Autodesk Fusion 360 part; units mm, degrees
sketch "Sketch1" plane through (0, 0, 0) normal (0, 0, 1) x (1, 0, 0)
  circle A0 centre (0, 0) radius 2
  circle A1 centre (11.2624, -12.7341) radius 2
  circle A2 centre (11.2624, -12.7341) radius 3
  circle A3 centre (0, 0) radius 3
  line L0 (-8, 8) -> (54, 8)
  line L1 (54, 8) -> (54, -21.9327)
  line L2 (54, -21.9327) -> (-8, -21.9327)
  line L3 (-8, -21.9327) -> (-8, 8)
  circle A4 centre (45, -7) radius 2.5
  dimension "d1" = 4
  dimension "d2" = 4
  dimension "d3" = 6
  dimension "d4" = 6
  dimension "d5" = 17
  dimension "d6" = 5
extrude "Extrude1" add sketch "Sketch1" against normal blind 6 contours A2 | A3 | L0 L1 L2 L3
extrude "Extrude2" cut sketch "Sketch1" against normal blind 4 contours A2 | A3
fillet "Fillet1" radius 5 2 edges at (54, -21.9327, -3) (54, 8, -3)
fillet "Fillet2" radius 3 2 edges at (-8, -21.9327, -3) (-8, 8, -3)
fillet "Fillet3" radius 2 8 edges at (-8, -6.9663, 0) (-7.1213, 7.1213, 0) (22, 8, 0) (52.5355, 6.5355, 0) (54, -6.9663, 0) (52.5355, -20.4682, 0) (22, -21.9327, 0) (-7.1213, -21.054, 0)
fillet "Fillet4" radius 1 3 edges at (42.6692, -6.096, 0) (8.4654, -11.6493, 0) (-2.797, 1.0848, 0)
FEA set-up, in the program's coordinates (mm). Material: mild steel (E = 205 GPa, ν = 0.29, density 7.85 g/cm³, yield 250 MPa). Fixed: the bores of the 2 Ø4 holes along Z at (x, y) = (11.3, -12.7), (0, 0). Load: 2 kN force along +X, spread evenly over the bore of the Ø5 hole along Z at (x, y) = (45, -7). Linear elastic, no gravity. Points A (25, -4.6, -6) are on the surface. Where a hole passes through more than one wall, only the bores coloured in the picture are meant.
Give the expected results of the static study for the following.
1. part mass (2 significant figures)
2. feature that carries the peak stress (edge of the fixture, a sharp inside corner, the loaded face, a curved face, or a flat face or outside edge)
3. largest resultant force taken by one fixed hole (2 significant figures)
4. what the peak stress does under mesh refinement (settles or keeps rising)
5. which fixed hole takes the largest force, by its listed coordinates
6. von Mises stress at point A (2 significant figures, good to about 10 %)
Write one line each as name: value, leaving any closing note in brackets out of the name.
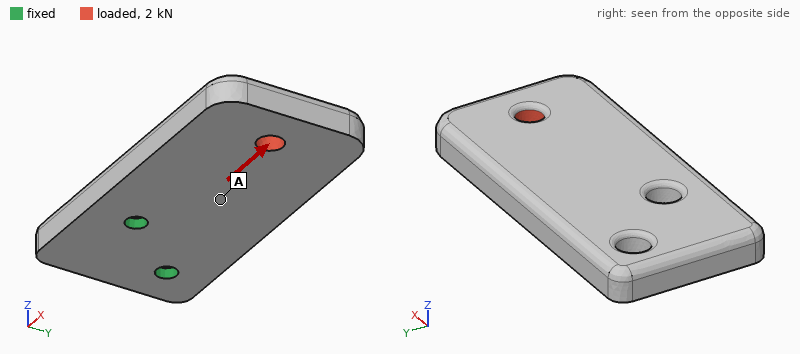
part mass: 82 g
feature that carries the peak stress: edge of the fixture
largest resultant force taken by one fixed hole: 1.1 kN
what the peak stress does under mesh refinement: keeps rising
which fixed hole takes the largest force, by its listed coordinates: (11.3, -12.7)
von Mises stress at point A: 18 MPa
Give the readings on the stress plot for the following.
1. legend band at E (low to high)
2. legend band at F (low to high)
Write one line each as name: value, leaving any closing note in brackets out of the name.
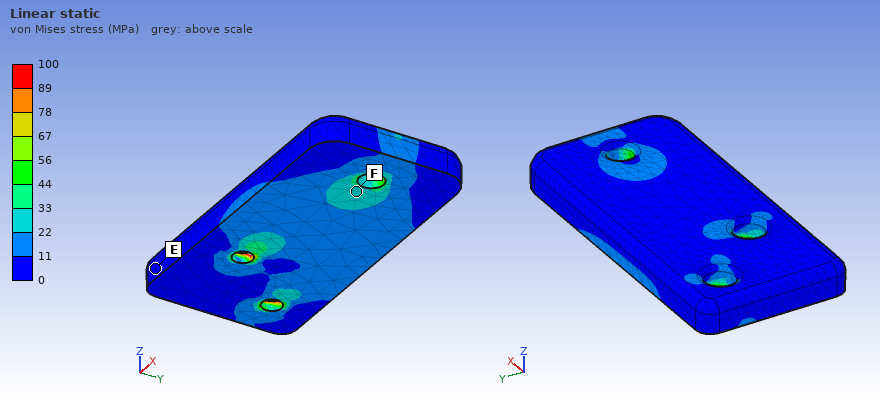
legend band at E: 0 to 11 MPa
legend band at F: 22 to 33 MPa
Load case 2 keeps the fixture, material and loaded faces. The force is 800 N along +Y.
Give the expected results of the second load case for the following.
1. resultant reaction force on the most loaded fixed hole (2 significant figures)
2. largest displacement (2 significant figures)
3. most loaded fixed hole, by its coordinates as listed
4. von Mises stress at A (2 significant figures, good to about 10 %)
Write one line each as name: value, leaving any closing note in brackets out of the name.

resultant reaction force on the most loaded fixed hole: 1.9 kN
largest displacement: 21 µm
most loaded fixed hole, by its coordinates as listed: (11.3, -12.7)
von Mises stress at A: 15 MPa
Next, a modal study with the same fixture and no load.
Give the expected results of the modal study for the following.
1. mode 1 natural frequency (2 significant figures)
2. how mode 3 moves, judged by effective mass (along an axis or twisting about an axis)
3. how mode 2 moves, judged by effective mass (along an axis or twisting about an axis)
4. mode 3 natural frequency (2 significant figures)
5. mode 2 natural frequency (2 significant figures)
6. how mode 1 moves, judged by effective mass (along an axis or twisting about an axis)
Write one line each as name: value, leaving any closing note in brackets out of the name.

mode 1 natural frequency: 1800 Hz
how mode 3 moves, judged by effective mass: along Y
how mode 2 moves, judged by effective mass: twisting about X
mode 3 natural frequency: 6700 Hz
mode 2 natural frequency: 5900 Hz
how mode 1 moves, judged by effective mass: along Z
